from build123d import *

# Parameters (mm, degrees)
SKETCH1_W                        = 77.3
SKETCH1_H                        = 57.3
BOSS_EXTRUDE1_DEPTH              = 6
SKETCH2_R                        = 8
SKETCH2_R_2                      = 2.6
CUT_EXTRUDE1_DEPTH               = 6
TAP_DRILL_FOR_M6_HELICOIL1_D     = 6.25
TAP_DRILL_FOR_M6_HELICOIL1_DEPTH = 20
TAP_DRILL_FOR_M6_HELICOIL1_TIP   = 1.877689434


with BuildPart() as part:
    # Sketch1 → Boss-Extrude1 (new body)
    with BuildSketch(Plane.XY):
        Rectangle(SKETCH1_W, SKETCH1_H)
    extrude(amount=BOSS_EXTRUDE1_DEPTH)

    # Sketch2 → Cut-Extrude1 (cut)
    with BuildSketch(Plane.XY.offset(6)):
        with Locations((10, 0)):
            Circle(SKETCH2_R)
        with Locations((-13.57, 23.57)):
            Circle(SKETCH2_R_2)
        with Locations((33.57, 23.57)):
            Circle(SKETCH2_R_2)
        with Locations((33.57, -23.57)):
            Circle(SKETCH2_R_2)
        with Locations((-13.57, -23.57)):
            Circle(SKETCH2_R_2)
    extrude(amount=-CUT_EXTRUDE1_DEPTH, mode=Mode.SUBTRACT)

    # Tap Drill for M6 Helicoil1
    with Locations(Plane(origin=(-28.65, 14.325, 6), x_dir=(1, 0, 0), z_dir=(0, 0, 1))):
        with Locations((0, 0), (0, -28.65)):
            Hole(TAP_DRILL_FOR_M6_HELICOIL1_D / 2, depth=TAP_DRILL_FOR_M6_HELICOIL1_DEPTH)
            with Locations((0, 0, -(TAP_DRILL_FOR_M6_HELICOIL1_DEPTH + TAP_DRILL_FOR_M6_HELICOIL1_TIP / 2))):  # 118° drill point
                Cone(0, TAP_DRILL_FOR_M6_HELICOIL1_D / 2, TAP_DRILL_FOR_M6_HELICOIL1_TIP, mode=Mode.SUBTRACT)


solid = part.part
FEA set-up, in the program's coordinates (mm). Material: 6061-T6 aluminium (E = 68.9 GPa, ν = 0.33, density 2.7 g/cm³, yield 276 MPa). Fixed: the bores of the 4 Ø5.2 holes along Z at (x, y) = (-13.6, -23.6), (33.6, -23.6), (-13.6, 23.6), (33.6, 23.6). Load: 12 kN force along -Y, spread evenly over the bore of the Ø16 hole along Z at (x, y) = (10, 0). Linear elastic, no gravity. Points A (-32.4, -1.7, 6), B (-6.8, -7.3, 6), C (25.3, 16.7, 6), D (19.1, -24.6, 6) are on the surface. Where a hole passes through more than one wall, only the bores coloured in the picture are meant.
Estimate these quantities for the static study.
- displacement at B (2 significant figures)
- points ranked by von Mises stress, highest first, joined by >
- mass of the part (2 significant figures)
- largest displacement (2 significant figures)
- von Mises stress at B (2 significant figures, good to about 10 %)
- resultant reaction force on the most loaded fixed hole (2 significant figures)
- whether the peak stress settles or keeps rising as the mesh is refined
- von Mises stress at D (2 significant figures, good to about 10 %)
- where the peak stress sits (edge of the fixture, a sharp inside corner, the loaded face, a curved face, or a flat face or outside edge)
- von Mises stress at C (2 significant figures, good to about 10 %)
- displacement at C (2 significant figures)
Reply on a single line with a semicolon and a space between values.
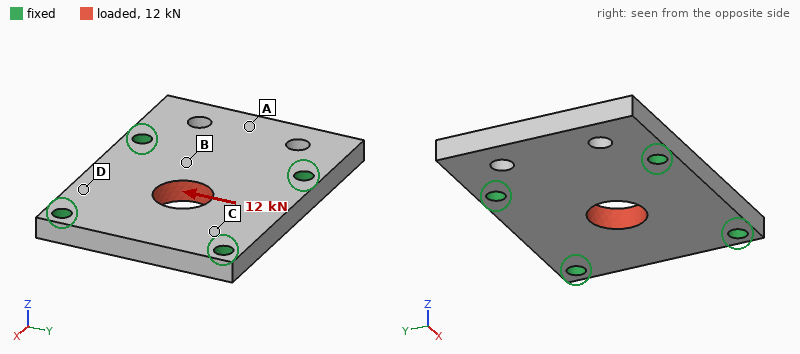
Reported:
8.1 µm; C > B > D > A; 66 g; 20 µm; 30 MPa; 3.4 kN; keeps rising; 15 MPa; edge of the fixture; 40 MPa; 8.0 µm
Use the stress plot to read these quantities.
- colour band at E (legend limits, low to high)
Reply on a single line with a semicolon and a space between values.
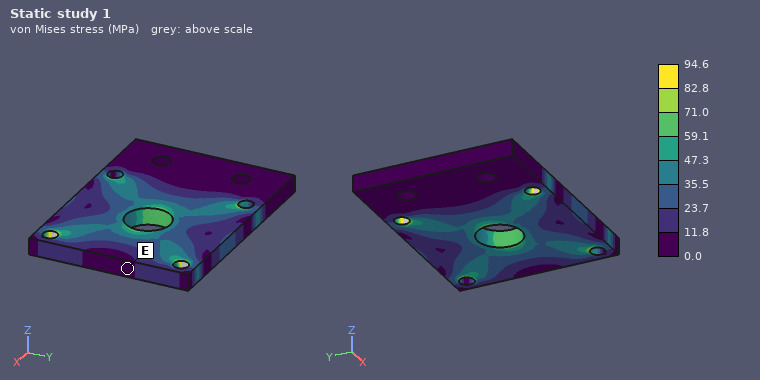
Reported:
0.0 to 11.8 MPa
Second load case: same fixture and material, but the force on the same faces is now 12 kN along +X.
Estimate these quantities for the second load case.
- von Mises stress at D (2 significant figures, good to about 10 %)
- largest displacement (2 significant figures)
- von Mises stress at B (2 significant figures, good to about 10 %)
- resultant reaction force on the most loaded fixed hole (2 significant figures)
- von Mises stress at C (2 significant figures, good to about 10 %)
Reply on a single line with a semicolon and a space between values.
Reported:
13 MPa; 20 µm; 26 MPa; 3.4 kN; 36 MPa
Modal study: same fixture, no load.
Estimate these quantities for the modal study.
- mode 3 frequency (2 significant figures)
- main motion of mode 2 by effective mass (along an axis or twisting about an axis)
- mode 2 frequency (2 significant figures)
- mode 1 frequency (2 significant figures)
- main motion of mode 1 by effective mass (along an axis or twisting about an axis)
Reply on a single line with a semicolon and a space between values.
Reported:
11 kHz; along Z; 9600 Hz; 6200 Hz; along Z
